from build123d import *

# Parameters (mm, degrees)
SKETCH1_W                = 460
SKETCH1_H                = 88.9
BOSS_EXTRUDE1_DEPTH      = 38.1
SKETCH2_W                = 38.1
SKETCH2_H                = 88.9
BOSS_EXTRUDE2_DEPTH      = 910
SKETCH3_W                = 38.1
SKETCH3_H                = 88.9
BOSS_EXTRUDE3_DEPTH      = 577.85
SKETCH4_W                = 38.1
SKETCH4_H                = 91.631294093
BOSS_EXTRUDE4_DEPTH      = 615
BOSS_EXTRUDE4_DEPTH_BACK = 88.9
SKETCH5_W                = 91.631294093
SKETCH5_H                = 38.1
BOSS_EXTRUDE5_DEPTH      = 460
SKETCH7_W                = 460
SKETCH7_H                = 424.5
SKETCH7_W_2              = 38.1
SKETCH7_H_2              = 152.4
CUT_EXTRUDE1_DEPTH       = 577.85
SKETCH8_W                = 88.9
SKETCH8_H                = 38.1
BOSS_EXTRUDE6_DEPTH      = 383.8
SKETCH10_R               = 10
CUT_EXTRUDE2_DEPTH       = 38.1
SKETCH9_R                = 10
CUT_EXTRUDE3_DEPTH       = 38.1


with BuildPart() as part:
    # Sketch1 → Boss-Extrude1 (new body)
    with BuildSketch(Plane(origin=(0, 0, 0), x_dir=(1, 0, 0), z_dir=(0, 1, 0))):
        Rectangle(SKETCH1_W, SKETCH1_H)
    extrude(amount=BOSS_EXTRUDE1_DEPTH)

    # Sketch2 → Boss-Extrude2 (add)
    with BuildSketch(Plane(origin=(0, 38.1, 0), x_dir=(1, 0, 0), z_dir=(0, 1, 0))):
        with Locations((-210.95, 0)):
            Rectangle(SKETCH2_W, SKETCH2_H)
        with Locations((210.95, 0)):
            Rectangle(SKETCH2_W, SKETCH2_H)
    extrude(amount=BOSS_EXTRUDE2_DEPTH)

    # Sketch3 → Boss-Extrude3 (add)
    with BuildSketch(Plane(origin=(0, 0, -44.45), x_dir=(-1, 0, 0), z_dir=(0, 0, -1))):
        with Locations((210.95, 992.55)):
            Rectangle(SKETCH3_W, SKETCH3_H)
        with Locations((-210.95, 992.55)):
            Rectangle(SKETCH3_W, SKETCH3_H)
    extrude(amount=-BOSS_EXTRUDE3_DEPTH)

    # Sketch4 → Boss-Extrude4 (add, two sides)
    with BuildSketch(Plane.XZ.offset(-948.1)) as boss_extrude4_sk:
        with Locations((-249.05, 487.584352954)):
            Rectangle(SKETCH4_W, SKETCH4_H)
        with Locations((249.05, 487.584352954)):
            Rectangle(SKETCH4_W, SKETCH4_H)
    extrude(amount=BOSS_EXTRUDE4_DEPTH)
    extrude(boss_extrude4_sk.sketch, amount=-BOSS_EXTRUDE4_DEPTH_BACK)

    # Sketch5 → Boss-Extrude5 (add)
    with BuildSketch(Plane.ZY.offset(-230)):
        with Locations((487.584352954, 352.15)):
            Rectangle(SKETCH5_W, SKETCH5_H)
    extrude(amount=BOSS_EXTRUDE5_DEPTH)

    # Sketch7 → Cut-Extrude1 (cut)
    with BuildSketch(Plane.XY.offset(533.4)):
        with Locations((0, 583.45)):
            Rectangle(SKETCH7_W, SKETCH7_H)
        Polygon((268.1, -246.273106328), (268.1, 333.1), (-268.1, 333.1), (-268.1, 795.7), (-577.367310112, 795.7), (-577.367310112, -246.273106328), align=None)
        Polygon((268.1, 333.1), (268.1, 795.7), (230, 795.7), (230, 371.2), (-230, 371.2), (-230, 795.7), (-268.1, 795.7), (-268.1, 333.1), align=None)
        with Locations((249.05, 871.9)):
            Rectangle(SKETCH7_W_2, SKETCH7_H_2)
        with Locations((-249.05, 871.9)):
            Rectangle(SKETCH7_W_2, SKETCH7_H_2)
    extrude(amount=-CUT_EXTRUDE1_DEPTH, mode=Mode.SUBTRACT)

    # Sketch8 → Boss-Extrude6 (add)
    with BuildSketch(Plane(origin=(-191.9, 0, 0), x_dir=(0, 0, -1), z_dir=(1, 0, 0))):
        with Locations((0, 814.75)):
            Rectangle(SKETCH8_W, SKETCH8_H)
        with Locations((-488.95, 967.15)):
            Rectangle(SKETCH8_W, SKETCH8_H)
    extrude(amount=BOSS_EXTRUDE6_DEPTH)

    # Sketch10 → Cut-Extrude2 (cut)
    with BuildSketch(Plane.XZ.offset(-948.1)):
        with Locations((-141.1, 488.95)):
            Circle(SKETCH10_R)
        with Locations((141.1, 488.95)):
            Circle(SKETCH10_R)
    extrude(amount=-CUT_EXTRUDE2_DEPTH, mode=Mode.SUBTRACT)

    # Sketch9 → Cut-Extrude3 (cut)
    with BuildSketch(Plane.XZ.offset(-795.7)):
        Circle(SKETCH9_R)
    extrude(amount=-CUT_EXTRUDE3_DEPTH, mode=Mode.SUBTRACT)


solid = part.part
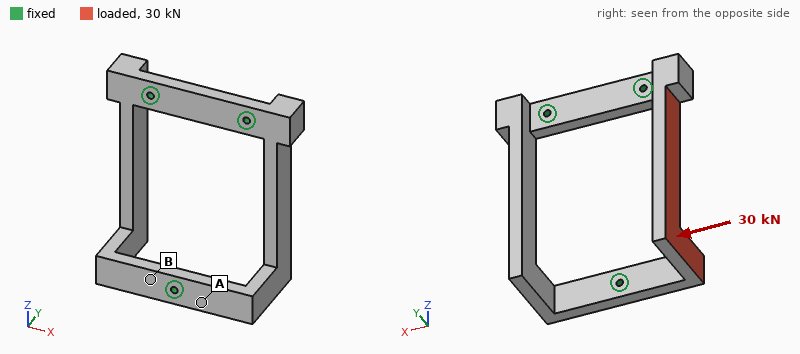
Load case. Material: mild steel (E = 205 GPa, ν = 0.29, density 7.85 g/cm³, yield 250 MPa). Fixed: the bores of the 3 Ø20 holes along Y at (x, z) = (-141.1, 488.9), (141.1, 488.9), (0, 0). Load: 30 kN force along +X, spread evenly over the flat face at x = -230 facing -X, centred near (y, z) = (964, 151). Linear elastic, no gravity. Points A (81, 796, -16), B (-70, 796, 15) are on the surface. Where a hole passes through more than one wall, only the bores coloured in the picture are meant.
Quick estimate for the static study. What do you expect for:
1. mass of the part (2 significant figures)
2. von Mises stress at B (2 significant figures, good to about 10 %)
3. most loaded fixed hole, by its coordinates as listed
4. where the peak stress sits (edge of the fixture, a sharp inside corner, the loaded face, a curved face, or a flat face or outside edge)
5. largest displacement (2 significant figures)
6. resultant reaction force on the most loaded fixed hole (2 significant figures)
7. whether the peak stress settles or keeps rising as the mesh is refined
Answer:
64 kg
50 MPa
(0, 0)
edge of the fixture
0.90 mm
17 kN
keeps rising
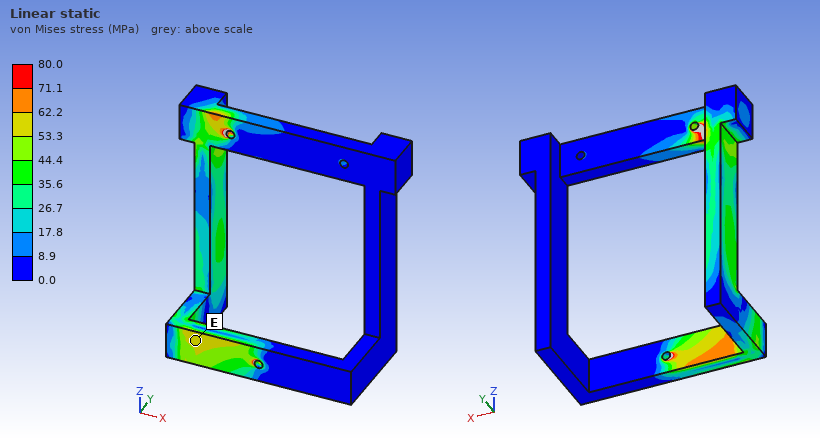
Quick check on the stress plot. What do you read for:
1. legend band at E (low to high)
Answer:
53.3 to 62.2 MPa
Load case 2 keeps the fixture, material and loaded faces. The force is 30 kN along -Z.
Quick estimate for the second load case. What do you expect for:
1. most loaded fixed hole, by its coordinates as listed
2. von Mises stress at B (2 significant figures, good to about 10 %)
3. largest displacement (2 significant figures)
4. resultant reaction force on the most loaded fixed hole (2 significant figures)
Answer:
(-141.1, 488.9)
9.6 MPa
0.11 mm
30 kN
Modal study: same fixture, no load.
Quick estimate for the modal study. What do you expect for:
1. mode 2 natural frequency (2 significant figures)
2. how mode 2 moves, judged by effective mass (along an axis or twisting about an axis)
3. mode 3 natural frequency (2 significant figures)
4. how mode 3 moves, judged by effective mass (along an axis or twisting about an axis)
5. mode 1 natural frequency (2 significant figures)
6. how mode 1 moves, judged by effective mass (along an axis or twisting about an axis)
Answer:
250 Hz
along Y
470 Hz
along X
240 Hz
along X
